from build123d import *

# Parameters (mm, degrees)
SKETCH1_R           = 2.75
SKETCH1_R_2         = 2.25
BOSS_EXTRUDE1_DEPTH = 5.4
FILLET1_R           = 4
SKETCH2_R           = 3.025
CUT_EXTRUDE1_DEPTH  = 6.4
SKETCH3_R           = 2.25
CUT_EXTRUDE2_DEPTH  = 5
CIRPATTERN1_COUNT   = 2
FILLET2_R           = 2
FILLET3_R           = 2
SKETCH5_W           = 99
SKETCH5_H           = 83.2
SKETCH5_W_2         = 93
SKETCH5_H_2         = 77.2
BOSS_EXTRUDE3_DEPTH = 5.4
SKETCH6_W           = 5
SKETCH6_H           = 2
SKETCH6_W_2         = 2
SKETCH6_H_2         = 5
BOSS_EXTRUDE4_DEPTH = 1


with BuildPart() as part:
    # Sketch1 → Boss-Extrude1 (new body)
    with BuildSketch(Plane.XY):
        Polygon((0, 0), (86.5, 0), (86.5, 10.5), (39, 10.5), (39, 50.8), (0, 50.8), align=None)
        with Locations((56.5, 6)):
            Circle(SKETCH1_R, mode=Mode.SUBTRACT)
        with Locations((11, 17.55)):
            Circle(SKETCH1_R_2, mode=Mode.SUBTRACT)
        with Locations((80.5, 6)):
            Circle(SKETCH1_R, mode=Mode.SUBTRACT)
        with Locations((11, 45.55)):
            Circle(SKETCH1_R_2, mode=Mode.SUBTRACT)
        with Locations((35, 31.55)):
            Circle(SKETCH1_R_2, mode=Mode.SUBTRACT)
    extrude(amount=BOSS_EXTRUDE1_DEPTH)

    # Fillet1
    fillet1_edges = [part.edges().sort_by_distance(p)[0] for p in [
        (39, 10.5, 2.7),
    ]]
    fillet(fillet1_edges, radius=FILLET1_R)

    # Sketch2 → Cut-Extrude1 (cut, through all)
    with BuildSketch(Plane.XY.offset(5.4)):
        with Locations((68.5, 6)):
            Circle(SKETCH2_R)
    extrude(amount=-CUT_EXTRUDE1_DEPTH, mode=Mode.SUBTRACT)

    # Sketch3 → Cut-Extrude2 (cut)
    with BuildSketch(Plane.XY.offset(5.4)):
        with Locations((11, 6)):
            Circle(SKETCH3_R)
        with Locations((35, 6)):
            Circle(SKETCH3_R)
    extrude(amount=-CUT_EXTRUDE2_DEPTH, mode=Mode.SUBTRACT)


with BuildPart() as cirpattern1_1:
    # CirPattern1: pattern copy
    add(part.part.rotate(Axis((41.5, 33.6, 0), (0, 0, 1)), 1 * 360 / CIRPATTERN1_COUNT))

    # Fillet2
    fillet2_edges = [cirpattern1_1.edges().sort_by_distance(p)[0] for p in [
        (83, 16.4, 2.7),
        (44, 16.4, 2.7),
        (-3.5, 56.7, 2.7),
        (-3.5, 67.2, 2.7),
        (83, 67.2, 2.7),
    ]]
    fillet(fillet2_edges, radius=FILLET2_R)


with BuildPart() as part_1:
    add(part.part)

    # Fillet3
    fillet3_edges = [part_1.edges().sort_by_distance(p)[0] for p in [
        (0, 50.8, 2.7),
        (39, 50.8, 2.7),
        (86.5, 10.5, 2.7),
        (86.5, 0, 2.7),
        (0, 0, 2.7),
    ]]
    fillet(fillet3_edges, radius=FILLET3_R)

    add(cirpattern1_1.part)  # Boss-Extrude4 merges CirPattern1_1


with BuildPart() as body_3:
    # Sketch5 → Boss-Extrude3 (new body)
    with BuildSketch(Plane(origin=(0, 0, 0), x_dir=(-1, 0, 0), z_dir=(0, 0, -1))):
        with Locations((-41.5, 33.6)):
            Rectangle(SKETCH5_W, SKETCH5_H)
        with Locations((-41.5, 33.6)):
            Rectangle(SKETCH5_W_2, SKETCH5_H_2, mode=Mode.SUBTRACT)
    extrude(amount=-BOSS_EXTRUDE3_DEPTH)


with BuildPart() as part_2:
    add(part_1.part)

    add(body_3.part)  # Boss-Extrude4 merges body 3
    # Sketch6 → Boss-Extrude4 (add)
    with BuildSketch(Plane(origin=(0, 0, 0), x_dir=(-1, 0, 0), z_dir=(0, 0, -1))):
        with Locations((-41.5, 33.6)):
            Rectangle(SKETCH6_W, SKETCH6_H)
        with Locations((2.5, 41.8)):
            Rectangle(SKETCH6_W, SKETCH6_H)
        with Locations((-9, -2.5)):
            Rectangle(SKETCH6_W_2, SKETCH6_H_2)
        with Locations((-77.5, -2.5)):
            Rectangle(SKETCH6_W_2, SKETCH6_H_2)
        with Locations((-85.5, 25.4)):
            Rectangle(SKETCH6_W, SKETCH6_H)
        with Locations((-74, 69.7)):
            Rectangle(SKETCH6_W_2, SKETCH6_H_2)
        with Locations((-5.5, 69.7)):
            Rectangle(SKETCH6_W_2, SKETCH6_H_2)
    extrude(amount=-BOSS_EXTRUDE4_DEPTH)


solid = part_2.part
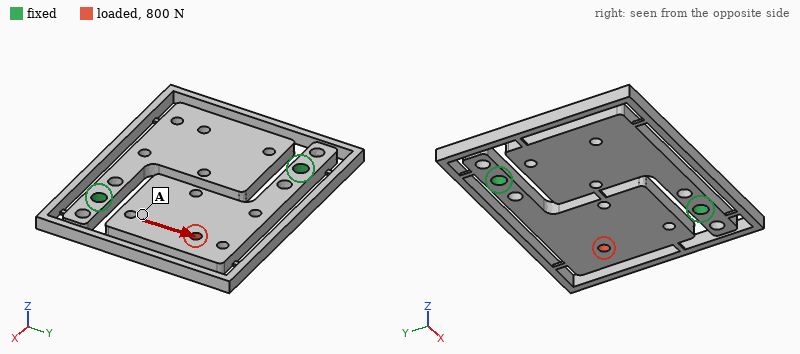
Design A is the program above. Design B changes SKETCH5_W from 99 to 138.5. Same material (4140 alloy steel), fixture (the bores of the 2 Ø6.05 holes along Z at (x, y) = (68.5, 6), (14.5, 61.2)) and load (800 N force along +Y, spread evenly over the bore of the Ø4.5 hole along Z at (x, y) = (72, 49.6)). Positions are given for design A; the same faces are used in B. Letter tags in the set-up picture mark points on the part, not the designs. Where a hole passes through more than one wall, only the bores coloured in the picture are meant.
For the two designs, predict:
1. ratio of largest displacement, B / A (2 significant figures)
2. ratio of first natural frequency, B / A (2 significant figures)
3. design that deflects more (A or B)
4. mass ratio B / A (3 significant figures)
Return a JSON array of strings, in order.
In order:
["0.65", "0.55", "A", "1.57"]
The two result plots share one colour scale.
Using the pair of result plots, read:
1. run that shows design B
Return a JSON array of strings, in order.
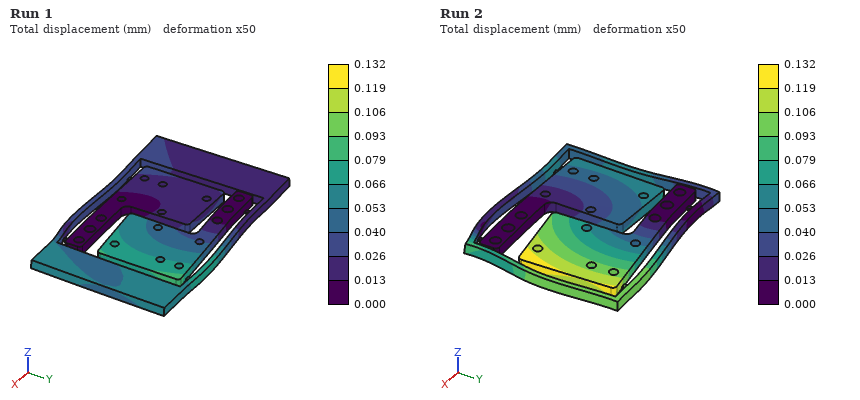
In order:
["Run 1"]
